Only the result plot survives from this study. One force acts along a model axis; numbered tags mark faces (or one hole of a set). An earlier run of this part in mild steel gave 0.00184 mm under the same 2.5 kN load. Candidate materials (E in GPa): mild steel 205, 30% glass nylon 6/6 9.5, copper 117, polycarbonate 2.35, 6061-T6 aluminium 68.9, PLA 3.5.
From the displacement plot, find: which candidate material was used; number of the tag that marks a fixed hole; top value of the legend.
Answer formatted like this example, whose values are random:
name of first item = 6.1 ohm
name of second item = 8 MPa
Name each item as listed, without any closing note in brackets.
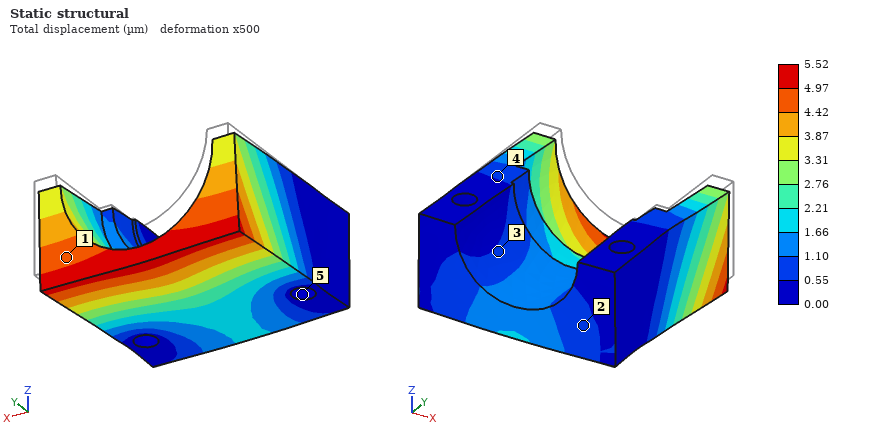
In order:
which candidate material was used = 6061-T6 aluminium
number of the tag that marks a fixed hole = 5
top value of the legend = 5.52 µm
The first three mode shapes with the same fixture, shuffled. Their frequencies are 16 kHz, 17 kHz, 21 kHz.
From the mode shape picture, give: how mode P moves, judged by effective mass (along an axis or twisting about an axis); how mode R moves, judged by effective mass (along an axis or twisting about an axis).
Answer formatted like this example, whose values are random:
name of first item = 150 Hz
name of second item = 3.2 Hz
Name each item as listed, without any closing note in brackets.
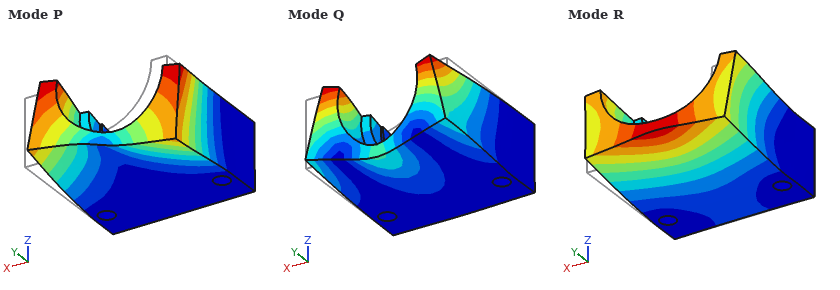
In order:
how mode P moves, judged by effective mass = along X
how mode R moves, judged by effective mass = along Z
